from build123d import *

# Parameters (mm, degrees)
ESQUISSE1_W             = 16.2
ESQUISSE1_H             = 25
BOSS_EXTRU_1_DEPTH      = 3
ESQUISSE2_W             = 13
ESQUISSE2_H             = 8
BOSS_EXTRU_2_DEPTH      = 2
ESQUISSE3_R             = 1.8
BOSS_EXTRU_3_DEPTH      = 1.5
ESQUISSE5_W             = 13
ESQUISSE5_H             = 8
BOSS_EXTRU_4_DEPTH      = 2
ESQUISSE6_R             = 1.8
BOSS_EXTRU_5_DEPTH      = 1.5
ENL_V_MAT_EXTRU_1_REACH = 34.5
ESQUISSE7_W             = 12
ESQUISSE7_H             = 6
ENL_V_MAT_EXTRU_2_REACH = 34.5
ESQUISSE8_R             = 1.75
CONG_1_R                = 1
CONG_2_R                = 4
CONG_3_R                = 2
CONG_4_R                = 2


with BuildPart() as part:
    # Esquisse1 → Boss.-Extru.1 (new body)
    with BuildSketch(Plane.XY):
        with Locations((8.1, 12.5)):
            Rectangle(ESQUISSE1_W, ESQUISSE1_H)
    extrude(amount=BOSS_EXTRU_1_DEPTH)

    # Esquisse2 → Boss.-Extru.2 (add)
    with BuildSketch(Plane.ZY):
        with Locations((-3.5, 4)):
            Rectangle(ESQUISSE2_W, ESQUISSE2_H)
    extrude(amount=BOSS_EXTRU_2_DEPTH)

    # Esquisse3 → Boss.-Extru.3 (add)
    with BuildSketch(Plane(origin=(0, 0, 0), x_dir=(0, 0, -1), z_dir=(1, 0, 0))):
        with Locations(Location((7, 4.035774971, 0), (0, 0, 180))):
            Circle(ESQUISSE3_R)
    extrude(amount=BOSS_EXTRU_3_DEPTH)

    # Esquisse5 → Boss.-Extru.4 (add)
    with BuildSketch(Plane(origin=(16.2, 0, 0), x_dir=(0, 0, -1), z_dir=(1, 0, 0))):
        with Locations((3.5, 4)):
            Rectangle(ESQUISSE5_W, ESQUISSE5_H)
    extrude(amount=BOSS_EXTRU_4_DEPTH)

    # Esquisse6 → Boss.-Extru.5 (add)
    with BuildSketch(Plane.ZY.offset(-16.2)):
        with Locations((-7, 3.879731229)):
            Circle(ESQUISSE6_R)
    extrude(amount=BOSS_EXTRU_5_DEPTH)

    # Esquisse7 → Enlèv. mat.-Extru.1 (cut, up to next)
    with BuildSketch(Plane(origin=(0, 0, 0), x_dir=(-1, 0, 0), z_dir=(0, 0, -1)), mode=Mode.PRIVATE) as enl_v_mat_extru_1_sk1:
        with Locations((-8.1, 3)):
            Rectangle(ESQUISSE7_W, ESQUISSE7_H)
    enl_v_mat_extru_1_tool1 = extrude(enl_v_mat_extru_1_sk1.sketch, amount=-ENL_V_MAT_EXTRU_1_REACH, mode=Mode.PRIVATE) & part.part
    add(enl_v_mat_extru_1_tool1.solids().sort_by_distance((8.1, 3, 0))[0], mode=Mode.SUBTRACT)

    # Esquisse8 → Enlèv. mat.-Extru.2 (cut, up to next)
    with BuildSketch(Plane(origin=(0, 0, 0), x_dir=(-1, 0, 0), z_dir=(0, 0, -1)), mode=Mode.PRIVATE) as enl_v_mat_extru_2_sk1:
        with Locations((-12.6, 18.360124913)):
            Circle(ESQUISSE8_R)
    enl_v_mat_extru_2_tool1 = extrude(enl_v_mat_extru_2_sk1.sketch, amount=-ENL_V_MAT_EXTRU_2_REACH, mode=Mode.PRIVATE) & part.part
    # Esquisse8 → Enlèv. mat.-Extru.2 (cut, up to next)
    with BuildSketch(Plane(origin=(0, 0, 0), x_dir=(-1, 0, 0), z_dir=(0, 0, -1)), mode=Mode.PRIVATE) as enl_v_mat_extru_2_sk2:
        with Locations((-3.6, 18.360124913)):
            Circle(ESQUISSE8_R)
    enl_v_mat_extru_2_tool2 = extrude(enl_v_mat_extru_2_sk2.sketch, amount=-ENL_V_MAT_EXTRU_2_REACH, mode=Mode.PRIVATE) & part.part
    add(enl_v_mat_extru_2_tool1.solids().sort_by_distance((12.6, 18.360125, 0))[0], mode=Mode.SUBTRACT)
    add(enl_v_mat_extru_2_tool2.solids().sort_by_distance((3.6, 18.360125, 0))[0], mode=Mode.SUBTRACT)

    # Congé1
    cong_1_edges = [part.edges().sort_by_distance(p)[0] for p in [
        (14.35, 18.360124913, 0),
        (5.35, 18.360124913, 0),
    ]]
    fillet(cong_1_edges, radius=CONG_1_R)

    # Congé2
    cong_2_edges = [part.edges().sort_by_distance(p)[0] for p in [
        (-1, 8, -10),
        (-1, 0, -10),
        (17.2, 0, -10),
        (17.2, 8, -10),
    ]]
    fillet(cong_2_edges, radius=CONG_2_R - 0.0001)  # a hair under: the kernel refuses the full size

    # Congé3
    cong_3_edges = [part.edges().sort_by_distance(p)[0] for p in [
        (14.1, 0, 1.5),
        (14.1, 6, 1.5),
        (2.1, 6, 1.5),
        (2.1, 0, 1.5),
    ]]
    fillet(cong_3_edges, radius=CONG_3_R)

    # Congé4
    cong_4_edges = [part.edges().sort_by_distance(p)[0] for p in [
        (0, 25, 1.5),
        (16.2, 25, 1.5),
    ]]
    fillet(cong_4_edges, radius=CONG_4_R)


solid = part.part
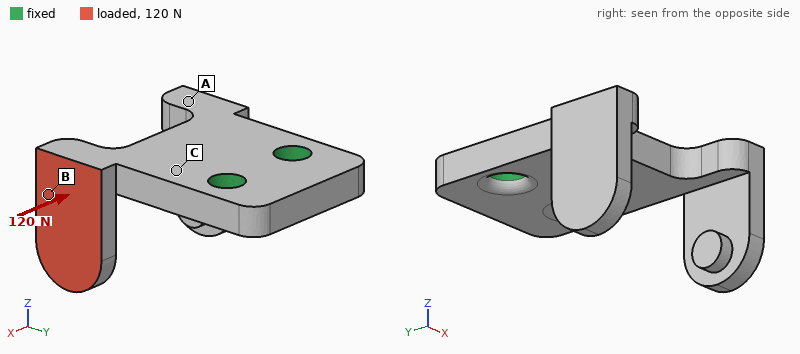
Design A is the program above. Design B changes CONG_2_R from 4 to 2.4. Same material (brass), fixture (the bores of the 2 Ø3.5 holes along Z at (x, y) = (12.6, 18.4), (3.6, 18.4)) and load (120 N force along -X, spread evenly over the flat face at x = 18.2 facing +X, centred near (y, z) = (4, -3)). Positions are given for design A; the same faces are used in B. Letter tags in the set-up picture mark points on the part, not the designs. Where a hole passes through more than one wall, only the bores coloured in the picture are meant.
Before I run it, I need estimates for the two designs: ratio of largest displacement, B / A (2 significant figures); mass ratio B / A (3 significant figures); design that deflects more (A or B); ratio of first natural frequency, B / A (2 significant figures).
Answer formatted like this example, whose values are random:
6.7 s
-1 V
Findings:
1.1
1.01
B
0.97
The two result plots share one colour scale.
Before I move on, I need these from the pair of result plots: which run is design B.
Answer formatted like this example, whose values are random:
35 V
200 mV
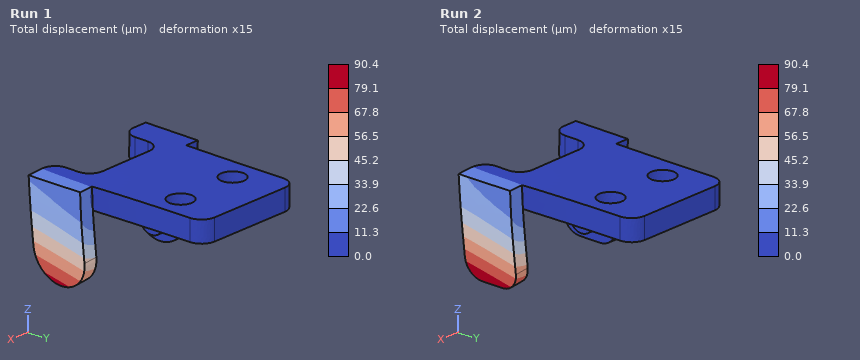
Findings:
Run 2
